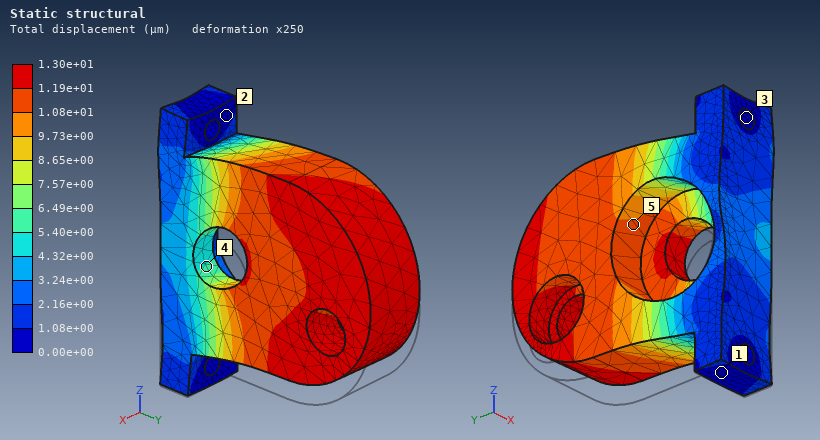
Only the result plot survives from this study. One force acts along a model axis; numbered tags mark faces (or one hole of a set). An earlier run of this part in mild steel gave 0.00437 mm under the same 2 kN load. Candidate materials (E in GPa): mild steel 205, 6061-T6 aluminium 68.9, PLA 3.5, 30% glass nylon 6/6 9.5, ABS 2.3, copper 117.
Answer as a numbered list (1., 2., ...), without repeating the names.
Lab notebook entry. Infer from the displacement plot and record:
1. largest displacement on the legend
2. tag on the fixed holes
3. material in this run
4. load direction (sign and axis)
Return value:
1. 1.30e+01 µm
2. 3
3. 6061-T6 aluminium
4. +Z
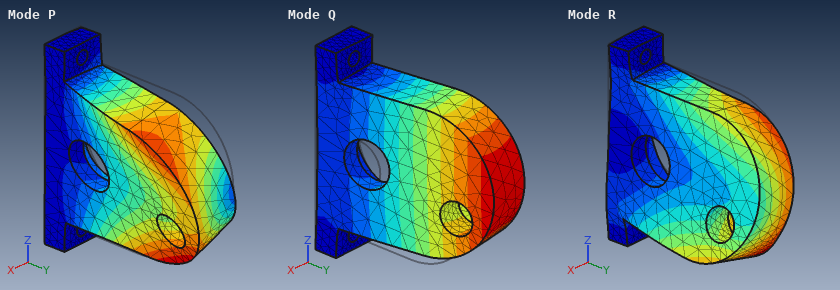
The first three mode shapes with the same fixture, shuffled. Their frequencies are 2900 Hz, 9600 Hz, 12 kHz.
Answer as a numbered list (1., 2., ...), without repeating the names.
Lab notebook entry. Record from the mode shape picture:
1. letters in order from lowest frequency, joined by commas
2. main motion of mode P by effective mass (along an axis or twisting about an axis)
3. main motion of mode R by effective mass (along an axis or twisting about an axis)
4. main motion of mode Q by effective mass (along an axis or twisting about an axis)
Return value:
1. Q, R, P
2. along Z
3. along Z
4. along X
